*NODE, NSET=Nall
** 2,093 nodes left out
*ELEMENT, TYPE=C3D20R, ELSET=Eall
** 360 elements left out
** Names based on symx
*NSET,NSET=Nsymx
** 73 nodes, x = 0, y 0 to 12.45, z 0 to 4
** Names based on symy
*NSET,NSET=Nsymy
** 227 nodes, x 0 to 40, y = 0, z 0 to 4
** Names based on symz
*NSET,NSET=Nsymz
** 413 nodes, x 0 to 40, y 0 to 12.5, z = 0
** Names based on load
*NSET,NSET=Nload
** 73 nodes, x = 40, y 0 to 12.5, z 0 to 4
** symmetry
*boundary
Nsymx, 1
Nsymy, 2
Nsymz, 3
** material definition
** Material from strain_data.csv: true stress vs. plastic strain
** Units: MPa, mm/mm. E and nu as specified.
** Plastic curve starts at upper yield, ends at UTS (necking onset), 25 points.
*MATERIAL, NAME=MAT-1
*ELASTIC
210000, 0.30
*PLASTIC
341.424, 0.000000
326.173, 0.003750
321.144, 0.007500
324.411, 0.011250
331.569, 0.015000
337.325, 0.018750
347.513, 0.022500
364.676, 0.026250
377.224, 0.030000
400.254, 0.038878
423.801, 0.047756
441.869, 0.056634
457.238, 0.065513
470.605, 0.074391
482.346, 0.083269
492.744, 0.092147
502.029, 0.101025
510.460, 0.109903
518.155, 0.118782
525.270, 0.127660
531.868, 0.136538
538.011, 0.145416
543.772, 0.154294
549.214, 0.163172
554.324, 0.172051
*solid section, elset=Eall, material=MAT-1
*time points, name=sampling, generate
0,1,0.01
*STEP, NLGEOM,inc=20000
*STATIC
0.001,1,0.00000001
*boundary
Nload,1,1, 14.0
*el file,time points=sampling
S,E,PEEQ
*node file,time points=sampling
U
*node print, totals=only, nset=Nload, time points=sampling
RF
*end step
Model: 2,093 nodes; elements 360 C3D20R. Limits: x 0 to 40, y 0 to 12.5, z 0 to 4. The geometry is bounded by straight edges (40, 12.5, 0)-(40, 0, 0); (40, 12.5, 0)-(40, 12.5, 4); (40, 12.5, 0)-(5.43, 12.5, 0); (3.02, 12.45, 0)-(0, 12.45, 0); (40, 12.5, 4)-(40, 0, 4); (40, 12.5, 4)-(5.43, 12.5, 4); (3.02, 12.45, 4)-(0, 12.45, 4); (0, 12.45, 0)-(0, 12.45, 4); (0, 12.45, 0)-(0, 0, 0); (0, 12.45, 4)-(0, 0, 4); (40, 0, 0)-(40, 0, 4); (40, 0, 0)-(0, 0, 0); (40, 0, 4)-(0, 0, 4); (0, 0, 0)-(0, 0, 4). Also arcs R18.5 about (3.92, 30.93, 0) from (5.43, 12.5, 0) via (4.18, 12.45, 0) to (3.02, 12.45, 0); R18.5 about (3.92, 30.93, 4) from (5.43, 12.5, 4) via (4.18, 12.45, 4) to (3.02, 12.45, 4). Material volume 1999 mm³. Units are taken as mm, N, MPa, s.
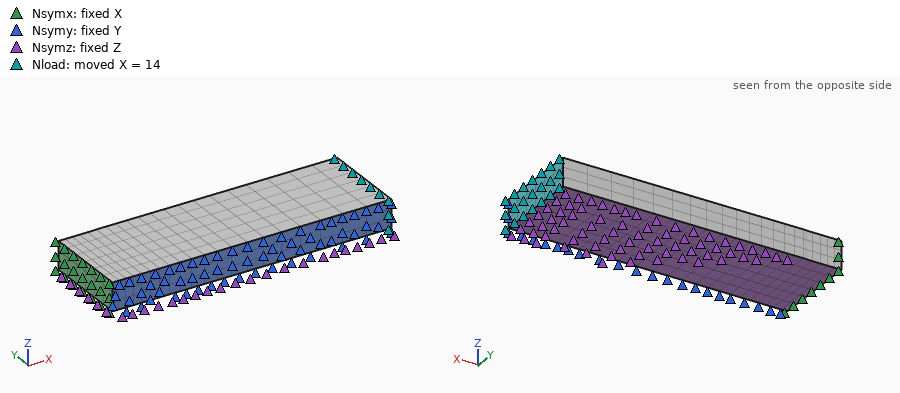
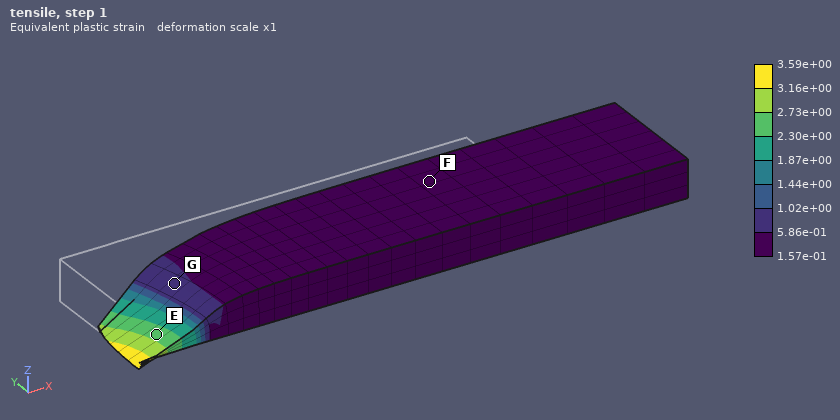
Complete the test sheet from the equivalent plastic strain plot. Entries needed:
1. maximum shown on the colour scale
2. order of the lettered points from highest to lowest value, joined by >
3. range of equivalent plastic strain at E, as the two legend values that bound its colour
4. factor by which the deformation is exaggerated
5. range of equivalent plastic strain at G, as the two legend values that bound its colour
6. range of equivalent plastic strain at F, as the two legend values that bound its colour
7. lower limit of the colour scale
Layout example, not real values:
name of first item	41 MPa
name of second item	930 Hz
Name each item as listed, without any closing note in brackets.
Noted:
maximum shown on the colour scale	3.59e+00
order of the lettered points from highest to lowest value, joined by >	E > G > F
range of equivalent plastic strain at E, as the two legend values that bound its colour	2.30e+00 to 2.73e+00
factor by which the deformation is exaggerated	1
range of equivalent plastic strain at G, as the two legend values that bound its colour	5.86e-01 to 1.02e+00
range of equivalent plastic strain at F, as the two legend values that bound its colour	1.57e-01 to 5.86e-01
lower limit of the colour scale	1.57e-01
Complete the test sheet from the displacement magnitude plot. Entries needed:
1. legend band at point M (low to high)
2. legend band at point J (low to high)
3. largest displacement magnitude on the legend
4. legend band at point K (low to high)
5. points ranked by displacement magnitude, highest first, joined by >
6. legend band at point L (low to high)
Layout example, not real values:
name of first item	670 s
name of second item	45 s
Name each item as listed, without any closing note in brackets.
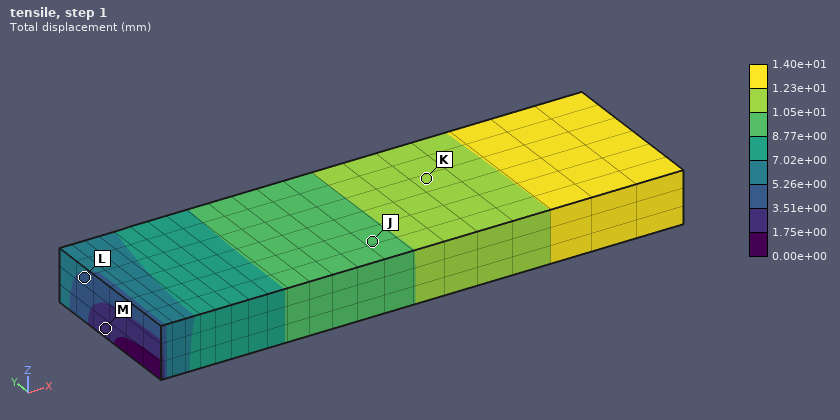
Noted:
legend band at point M	1.75e+00 to 3.51e+00 mm
legend band at point J	8.77e+00 to 1.05e+01 mm
largest displacement magnitude on the legend	1.40e+01 mm
legend band at point K	1.05e+01 to 1.23e+01 mm
points ranked by displacement magnitude, highest first, joined by >	K > J > L > M
legend band at point L	3.51e+00 to 5.26e+00 mm
